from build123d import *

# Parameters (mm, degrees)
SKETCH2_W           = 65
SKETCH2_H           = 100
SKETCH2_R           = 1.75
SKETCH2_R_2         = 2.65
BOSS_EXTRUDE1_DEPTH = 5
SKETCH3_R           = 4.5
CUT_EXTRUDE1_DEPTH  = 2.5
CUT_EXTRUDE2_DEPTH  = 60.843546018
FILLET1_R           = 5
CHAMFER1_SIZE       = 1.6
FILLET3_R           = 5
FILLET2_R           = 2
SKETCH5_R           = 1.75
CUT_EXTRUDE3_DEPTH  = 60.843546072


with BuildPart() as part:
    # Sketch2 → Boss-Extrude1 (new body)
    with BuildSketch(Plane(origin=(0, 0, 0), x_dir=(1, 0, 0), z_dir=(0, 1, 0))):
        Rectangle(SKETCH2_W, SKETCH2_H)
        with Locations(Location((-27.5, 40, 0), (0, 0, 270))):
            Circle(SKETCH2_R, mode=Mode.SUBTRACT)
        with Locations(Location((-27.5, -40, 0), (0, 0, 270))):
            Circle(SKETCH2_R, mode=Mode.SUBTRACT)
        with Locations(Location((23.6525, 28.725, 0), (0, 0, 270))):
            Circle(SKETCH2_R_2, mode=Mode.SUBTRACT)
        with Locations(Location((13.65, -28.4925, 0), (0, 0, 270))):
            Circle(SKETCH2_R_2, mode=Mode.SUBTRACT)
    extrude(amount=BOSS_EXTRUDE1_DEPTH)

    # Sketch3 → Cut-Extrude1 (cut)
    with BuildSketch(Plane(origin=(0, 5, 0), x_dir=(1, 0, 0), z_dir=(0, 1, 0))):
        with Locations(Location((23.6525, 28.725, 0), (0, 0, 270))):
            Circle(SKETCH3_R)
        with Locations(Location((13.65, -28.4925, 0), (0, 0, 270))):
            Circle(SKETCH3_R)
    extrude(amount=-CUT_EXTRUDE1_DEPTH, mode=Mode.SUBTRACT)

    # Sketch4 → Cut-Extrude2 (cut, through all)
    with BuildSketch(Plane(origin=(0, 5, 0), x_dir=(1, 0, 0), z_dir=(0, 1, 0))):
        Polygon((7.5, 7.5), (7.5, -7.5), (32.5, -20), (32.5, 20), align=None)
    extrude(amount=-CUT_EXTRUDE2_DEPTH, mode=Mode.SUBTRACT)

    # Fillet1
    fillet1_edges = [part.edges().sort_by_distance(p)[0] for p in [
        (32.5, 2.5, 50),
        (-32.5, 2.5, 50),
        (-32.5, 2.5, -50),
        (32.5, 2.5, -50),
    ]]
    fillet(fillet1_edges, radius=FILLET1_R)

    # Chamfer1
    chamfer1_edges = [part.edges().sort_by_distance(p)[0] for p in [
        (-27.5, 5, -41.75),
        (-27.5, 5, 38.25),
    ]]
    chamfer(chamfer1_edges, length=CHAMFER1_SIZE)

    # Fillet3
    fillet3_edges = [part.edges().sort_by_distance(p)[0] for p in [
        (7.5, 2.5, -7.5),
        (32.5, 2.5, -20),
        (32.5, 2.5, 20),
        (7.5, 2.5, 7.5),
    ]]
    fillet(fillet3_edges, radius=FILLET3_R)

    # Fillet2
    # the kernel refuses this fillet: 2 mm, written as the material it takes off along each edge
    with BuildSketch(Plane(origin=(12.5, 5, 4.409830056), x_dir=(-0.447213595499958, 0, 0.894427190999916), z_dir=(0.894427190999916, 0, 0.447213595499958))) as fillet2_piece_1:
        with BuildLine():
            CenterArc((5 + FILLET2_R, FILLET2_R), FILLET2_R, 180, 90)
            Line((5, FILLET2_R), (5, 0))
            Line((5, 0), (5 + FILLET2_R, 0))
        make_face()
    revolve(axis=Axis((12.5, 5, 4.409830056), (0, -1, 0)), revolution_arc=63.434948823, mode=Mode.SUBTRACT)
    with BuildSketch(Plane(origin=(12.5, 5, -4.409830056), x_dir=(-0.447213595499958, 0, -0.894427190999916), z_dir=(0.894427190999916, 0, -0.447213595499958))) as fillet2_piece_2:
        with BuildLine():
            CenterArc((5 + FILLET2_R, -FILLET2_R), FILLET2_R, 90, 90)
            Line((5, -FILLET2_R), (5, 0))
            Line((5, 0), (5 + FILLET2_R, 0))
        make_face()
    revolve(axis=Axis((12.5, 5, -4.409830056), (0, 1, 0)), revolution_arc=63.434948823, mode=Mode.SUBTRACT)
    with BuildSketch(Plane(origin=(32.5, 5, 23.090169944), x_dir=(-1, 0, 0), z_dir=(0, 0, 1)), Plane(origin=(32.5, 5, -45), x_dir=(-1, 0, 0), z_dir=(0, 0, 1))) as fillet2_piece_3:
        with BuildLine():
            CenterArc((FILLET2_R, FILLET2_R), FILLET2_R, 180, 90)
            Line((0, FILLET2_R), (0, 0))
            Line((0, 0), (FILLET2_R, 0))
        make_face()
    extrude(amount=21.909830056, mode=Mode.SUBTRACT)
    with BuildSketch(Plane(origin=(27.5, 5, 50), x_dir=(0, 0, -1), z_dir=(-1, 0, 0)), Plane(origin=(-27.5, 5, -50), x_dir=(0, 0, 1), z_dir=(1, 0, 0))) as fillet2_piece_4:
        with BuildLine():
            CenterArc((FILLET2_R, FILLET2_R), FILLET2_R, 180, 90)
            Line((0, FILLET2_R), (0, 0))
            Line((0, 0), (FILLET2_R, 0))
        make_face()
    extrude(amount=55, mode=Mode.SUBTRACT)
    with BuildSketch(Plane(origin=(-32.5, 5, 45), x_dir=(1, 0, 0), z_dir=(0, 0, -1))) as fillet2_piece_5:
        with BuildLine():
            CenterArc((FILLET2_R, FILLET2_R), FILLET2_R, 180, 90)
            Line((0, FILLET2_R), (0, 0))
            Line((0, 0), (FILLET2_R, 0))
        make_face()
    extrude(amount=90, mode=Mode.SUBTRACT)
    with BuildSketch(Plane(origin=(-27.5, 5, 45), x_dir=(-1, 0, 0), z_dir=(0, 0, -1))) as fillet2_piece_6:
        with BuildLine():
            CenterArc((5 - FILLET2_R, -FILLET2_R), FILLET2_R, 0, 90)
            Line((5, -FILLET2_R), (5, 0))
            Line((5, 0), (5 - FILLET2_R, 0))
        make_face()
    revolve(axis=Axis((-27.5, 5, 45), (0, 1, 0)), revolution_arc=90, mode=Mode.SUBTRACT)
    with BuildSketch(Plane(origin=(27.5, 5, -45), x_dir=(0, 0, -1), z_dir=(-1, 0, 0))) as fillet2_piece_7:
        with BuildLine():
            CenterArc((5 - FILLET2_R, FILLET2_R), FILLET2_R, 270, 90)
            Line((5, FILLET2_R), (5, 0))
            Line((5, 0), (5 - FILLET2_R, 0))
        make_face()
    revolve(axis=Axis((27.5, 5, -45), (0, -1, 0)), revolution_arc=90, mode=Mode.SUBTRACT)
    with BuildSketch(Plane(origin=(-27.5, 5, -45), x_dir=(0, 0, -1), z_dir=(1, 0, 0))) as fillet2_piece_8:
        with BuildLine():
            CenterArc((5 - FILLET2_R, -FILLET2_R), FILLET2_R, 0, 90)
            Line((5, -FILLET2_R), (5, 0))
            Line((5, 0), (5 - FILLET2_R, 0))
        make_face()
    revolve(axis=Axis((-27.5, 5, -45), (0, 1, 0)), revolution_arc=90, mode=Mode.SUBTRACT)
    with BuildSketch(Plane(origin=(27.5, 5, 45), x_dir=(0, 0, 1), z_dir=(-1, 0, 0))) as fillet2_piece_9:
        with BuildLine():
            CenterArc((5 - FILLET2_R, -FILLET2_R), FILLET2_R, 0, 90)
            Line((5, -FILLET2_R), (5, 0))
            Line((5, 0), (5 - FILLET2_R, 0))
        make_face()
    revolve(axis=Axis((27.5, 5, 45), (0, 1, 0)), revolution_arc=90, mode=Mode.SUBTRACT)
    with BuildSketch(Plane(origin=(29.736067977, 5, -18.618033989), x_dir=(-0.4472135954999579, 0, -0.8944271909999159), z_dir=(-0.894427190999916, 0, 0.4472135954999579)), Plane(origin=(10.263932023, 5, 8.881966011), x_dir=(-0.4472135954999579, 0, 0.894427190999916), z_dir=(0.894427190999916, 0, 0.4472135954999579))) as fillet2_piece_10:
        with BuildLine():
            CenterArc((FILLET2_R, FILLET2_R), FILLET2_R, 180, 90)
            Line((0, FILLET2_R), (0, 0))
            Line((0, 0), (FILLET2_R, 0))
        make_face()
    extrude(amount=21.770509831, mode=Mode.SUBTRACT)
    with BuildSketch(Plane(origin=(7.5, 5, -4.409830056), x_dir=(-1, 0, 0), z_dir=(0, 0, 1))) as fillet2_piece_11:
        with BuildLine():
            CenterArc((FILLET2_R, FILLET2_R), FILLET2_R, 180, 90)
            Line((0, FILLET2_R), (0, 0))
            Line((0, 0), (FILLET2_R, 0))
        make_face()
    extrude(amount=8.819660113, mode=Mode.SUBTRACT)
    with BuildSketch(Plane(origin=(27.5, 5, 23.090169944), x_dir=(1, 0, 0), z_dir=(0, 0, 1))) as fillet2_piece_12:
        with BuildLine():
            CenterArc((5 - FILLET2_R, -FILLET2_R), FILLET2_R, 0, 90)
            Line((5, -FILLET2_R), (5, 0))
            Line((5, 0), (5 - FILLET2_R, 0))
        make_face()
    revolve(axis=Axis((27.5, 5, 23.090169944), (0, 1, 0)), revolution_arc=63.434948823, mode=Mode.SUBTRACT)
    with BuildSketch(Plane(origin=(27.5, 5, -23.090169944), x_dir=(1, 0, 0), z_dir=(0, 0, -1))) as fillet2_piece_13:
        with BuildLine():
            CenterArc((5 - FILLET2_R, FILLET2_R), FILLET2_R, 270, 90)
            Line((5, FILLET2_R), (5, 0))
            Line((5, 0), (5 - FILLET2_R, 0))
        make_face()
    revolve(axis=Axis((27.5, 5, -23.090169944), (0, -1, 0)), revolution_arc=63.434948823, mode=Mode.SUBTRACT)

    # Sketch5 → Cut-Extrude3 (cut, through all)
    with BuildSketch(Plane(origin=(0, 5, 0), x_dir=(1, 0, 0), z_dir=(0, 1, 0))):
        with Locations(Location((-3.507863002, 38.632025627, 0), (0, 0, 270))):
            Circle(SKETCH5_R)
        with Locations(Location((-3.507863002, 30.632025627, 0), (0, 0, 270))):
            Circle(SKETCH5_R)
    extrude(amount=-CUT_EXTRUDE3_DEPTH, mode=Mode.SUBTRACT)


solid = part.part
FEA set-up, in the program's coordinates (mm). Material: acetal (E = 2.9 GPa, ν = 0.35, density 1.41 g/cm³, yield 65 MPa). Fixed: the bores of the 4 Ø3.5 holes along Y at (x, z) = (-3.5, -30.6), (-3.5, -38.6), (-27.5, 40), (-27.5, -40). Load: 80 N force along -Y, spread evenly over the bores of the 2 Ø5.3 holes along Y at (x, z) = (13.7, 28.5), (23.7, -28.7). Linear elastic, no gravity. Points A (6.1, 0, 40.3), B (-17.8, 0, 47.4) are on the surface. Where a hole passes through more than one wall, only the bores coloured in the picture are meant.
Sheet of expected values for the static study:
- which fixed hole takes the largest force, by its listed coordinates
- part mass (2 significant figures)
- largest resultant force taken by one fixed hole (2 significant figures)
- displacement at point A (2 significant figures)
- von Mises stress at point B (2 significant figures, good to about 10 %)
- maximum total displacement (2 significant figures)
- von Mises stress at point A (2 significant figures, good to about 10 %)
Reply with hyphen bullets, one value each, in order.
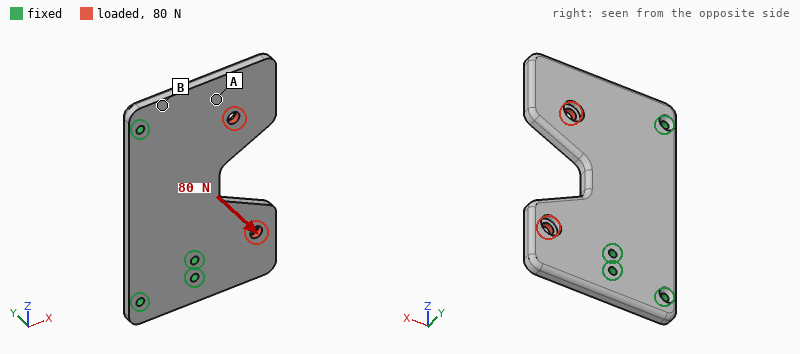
- (-3.5, -30.6)
- 39 g
- 91 N
- 0.60 mm
- 5.7 MPa
- 1.3 mm
- 1.5 MPa
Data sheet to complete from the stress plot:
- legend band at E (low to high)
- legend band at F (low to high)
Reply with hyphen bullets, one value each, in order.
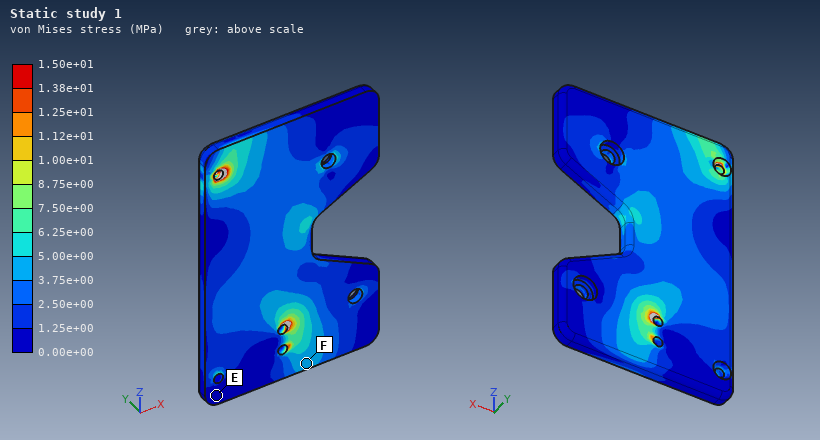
- 0.00e+00 to 1.25e+00 MPa
- 3.75e+00 to 5.00e+00 MPa
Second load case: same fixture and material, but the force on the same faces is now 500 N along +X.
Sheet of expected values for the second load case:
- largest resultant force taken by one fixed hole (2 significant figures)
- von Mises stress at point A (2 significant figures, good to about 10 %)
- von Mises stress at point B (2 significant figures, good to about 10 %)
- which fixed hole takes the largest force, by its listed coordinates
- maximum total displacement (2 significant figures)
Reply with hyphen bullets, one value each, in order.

- 220 N
- 2.4 MPa
- 2.9 MPa
- (-27.5, 40)
- 0.33 mm
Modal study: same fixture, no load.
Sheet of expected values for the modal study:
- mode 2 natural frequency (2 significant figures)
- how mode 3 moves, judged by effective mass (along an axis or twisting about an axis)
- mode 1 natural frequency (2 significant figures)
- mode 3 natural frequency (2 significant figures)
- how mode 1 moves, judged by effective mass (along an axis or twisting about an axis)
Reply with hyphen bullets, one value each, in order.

- 1000 Hz
- along Y
- 360 Hz
- 1100 Hz
- along Y
